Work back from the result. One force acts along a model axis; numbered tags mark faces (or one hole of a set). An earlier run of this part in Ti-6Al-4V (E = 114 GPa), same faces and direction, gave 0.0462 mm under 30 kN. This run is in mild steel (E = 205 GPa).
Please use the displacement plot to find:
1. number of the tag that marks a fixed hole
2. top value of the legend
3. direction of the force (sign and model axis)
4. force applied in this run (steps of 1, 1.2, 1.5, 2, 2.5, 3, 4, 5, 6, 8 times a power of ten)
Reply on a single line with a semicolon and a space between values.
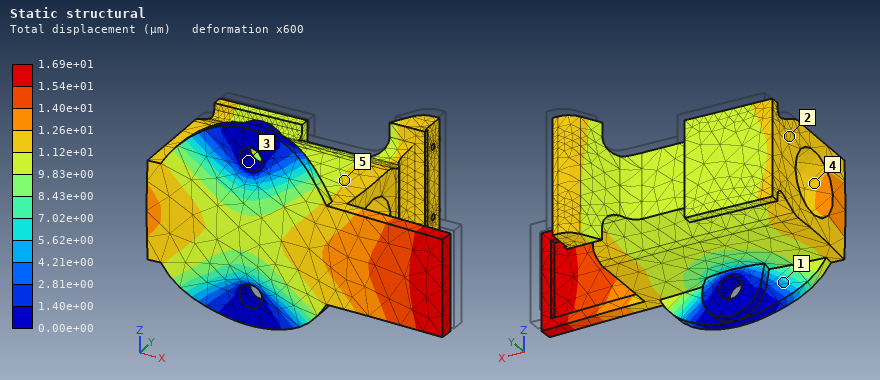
3; 1.69e+01 µm; -Y; 20 kN
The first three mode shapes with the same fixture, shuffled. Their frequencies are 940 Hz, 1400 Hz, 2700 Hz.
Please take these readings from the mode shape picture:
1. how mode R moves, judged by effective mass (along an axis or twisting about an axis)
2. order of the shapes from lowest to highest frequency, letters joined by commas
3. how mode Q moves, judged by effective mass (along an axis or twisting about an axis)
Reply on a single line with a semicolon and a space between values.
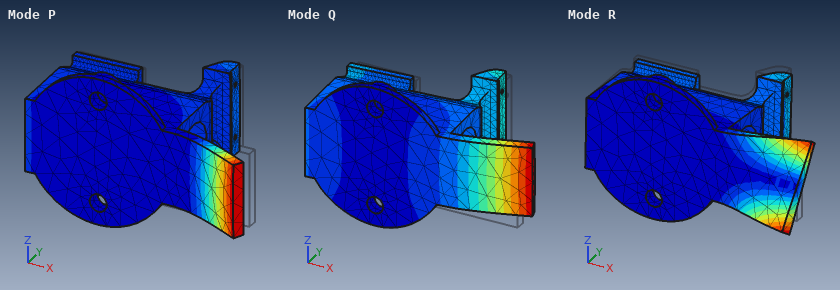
along Z; Q, P, R; along X
